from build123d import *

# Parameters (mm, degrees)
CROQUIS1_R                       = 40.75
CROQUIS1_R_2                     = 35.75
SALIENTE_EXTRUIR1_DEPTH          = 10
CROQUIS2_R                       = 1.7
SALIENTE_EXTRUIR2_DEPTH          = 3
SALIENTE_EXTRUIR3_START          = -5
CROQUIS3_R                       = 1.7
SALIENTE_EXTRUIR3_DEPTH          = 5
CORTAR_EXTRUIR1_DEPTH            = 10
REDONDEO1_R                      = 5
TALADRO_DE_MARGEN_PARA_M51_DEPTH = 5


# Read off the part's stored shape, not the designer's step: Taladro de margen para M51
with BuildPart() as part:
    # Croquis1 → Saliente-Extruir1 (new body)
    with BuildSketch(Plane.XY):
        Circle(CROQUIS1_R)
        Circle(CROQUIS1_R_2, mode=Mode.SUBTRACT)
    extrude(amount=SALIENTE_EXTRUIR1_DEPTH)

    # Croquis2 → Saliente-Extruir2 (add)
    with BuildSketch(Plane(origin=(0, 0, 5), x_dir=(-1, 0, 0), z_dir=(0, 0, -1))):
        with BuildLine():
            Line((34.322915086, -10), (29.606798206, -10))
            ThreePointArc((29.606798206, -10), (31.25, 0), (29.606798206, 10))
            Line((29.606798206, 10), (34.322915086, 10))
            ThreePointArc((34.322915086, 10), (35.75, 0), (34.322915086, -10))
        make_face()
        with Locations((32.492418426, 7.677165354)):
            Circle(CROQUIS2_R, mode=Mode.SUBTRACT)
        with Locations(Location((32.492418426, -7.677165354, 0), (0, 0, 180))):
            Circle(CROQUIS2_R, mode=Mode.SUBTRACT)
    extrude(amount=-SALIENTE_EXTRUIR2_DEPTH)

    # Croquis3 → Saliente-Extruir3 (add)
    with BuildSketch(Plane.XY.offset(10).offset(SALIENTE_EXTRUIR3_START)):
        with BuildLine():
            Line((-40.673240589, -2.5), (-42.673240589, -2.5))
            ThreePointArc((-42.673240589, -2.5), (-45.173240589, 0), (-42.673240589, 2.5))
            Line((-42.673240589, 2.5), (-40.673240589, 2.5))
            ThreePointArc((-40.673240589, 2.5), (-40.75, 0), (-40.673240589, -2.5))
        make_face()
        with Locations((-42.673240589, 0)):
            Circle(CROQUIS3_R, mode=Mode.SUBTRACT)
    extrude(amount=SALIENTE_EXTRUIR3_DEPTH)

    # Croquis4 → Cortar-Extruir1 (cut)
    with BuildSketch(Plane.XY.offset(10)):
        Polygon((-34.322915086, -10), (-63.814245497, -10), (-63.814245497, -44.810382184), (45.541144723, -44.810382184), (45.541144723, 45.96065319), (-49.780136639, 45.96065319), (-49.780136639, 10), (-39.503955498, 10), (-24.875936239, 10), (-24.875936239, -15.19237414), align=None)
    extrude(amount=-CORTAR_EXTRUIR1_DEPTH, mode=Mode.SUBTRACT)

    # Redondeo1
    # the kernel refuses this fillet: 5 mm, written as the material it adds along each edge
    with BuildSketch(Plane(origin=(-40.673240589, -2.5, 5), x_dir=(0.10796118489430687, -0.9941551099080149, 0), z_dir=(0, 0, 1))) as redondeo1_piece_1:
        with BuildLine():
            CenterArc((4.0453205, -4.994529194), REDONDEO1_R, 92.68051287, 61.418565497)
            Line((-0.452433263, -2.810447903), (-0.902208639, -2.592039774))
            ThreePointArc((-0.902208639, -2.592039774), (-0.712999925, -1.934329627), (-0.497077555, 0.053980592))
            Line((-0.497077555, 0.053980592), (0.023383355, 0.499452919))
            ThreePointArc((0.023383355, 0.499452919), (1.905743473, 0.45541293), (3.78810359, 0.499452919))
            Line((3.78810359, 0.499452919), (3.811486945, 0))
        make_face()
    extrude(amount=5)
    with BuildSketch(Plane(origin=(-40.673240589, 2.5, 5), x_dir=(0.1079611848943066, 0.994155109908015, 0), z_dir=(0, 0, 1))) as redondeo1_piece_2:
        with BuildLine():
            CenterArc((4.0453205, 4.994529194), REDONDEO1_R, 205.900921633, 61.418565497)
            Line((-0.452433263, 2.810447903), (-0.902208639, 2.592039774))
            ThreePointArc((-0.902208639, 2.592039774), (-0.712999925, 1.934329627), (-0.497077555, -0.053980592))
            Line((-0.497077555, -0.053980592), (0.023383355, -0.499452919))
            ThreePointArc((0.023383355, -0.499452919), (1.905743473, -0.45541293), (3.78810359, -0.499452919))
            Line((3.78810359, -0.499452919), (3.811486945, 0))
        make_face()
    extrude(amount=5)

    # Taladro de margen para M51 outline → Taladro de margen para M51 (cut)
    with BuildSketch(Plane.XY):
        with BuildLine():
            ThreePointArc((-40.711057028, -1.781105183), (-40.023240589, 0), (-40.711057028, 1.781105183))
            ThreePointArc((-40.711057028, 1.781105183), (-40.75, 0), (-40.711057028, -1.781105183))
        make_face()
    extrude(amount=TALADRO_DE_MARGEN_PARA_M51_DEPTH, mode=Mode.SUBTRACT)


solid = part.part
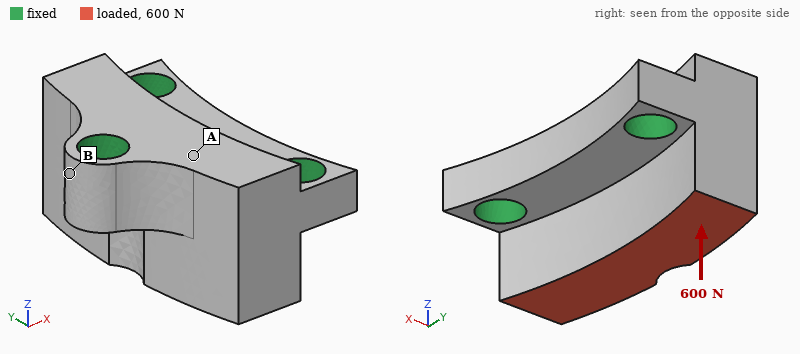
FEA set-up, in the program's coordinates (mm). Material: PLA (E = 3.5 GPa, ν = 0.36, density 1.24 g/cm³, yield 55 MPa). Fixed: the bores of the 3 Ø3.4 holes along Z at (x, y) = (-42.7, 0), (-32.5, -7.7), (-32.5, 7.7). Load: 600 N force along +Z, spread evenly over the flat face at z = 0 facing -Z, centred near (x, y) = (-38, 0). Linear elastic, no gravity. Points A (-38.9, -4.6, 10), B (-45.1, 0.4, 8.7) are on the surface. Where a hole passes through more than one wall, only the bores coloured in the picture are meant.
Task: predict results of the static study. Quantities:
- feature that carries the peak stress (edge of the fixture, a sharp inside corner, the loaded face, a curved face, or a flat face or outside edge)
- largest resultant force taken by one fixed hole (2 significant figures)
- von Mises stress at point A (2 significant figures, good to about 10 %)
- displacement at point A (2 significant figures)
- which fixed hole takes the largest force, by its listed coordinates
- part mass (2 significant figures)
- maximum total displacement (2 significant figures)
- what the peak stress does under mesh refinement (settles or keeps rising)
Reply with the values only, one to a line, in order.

edge of the fixture
310 N
8.8 MPa
21 µm
(-42.7, 0)
1.6 g
47 µm
keeps rising
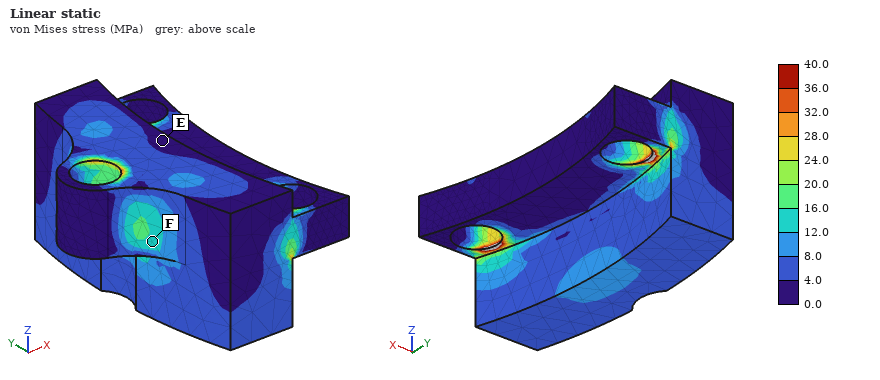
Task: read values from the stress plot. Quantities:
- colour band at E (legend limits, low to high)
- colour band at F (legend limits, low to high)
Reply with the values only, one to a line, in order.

0.0 to 4.0 MPa
12.0 to 16.0 MPa
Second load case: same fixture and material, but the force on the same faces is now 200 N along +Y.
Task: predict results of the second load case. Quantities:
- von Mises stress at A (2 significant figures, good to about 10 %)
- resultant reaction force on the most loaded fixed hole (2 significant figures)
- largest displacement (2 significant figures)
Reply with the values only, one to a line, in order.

4.2 MPa
93 N
48 µm
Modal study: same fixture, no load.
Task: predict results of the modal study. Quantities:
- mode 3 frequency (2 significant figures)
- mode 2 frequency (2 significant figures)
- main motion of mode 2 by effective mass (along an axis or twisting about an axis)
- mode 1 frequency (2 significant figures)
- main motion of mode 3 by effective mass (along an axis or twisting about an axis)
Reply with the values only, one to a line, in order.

23 kHz
18 kHz
along X
16 kHz
along Z
